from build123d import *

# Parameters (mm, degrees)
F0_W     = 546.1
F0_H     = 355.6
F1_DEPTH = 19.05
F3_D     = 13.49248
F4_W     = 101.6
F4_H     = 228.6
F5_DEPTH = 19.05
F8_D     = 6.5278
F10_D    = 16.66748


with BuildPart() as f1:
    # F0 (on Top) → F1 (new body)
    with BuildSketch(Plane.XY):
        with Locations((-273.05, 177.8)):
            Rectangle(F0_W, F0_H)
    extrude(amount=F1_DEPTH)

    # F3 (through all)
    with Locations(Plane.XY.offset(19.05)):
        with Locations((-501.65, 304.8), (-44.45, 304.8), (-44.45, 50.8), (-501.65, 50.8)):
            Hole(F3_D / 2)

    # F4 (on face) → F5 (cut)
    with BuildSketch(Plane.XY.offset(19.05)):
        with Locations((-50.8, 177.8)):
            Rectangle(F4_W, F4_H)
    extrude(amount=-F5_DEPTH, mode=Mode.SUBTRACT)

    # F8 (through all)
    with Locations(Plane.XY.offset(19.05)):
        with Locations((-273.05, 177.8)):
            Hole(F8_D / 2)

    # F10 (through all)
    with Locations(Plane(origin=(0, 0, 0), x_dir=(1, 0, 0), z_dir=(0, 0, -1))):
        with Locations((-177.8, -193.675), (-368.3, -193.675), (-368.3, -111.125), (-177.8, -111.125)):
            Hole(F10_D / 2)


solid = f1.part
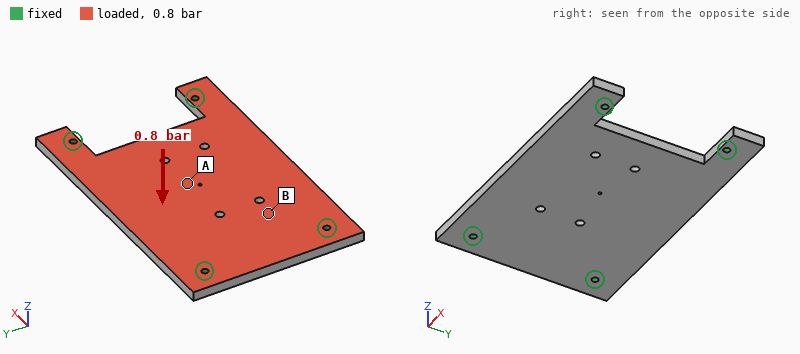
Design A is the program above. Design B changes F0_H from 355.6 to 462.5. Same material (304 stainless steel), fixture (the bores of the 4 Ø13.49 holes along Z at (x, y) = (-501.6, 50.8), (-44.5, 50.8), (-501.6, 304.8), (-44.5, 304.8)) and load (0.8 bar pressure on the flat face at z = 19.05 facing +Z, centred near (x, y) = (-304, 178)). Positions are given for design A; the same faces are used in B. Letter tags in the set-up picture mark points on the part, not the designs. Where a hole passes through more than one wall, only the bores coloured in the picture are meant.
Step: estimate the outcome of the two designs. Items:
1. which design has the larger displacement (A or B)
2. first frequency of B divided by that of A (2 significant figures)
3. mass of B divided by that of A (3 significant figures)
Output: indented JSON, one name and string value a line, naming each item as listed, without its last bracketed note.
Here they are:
{
  "which design has the larger displacement": "B",
  "first frequency of B divided by that of A": "0.97",
  "mass of B divided by that of A": "1.34"
}
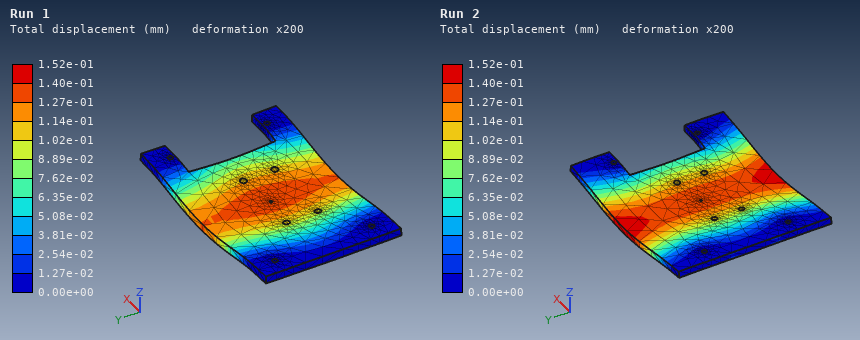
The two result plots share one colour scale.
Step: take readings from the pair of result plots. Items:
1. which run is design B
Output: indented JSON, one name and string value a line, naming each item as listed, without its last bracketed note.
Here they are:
{
  "which run is design B": "Run 2"
}
